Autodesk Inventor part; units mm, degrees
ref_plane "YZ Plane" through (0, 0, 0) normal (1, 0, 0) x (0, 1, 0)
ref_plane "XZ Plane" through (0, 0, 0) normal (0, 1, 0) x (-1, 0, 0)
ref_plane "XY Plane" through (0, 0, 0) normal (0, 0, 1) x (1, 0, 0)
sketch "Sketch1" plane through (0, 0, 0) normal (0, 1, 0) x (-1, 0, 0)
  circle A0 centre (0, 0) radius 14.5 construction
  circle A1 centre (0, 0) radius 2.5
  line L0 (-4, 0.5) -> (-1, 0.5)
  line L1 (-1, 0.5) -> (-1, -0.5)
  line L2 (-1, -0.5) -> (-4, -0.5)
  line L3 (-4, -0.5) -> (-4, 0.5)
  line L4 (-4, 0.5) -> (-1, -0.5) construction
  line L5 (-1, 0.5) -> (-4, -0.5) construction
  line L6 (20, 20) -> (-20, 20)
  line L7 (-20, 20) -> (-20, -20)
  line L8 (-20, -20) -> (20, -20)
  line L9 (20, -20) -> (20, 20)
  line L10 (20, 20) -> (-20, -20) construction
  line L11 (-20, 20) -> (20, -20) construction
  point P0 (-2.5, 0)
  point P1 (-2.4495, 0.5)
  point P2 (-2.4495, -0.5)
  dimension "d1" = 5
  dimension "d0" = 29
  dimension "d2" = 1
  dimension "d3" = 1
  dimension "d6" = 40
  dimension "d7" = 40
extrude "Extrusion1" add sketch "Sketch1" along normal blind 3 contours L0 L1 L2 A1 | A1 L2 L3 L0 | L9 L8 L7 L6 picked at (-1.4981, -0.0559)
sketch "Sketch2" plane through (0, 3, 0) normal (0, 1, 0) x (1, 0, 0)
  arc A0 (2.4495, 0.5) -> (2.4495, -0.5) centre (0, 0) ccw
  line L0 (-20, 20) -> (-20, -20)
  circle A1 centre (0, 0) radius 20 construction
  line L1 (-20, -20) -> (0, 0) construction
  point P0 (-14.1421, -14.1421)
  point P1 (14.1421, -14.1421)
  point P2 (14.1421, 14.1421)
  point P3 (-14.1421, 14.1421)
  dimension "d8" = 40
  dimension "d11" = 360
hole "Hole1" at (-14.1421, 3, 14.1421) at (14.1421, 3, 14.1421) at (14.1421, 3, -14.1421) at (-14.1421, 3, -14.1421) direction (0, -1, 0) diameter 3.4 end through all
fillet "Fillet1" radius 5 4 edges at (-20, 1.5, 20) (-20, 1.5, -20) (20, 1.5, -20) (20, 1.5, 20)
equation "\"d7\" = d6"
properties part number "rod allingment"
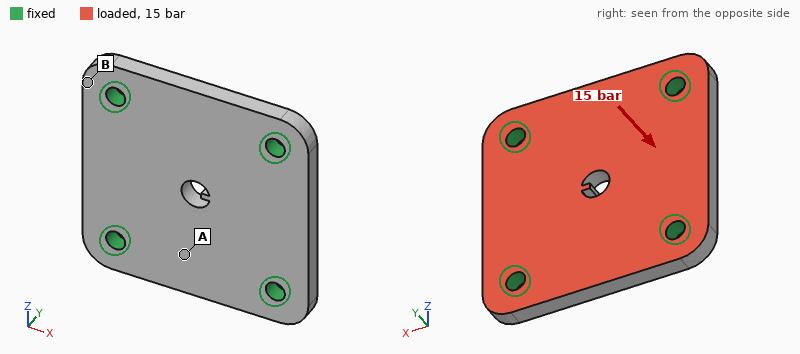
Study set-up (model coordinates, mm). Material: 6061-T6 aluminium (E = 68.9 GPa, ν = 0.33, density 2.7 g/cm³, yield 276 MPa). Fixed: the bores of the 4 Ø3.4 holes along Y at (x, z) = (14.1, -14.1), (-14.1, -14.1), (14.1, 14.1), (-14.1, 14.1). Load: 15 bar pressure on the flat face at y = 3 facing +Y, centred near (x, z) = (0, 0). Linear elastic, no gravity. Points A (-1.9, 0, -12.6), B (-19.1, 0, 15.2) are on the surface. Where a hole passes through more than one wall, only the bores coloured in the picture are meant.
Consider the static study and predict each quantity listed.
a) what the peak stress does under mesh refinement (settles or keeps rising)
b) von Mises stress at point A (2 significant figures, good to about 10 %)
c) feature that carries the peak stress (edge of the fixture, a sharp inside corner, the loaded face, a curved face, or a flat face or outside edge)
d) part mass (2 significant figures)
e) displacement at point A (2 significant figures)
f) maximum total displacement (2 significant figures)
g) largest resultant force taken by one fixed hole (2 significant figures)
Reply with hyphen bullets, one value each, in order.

- keeps rising
- 33 MPa
- edge of the fixture
- 12 g
- 21 µm
- 39 µm
- 570 N
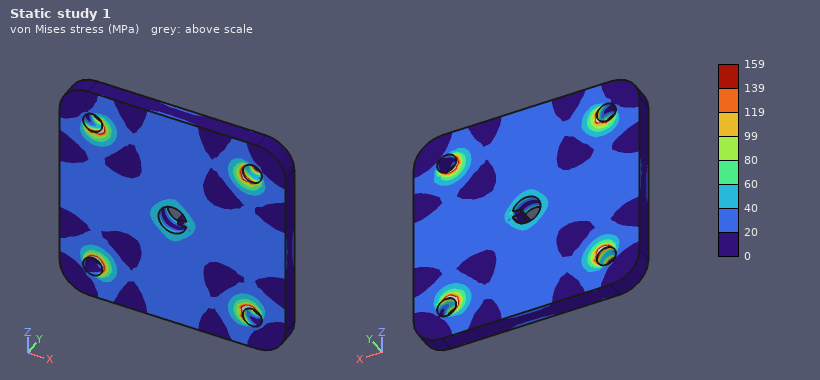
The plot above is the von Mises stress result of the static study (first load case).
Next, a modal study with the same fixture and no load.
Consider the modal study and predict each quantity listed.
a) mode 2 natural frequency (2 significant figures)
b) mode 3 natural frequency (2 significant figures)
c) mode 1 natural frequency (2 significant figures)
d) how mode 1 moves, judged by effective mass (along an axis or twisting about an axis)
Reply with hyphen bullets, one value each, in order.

- 21 kHz
- 21 kHz
- 14 kHz
- along Y
